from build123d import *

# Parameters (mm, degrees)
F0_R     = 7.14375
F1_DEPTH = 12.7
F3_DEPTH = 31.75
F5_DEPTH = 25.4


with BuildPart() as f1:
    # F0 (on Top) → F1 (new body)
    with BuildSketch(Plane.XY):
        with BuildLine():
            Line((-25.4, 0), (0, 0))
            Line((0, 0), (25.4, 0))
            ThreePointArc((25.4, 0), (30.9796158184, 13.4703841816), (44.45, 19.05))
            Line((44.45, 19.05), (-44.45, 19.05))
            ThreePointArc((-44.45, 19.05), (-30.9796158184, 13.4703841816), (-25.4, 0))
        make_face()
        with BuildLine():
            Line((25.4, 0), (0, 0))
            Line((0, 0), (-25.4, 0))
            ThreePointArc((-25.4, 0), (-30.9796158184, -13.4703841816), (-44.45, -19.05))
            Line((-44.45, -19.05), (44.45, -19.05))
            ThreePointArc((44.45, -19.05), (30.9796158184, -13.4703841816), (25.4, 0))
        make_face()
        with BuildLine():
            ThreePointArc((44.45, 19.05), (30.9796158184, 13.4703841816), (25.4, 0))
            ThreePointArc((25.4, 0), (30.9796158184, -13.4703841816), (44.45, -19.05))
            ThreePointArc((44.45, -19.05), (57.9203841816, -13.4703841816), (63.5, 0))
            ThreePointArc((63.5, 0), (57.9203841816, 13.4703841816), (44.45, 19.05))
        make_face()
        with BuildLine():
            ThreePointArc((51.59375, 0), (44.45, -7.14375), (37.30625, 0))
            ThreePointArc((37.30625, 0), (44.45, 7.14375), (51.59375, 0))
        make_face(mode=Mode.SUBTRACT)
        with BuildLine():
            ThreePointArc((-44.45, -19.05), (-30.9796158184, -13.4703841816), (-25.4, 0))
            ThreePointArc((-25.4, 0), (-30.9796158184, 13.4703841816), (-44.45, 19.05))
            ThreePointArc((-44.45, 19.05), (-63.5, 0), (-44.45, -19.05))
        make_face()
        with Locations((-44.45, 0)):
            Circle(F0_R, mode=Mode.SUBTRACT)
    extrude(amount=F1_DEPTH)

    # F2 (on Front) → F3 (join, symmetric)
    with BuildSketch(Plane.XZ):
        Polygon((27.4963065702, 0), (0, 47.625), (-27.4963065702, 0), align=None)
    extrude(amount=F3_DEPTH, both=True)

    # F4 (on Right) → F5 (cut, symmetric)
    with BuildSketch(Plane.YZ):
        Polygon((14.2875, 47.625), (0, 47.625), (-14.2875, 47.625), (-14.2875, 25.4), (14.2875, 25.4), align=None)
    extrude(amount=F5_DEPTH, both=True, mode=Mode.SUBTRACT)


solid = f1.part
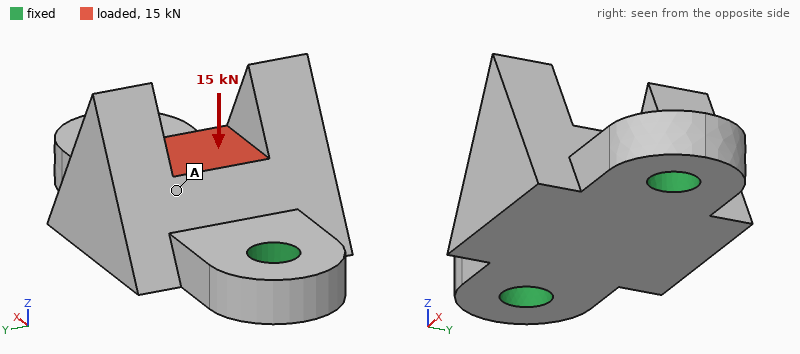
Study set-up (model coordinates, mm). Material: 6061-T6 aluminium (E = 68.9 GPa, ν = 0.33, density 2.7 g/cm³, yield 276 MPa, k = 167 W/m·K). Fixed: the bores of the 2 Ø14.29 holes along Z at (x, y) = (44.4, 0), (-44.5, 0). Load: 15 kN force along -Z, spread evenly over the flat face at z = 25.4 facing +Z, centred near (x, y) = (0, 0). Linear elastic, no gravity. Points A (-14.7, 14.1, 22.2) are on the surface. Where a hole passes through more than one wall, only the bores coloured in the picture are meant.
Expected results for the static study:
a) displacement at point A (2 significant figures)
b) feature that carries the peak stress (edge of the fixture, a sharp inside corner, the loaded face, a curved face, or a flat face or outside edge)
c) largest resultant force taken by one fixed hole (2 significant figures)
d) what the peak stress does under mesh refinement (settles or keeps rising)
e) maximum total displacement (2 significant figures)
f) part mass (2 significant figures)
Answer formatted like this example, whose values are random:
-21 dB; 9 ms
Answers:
45 µm; edge of the fixture; 8.0 kN; keeps rising; 50 µm; 280 g
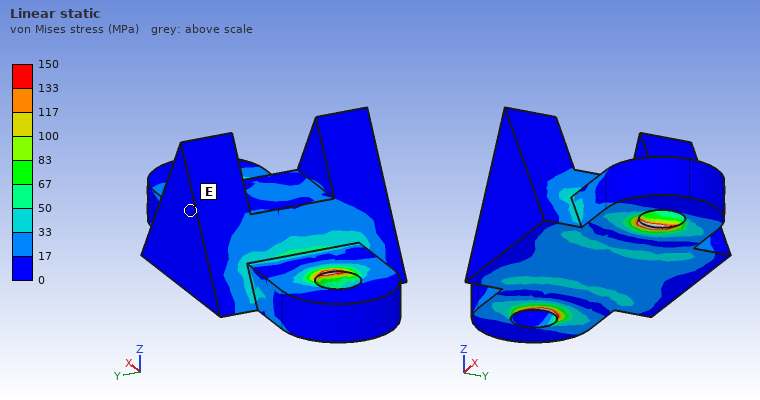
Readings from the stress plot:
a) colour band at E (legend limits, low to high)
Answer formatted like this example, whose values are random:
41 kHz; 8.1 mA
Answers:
0 to 17 MPa
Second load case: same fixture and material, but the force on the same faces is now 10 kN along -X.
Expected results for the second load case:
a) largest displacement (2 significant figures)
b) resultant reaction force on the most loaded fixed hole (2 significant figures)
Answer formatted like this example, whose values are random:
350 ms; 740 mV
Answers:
28 µm; 5.8 kN
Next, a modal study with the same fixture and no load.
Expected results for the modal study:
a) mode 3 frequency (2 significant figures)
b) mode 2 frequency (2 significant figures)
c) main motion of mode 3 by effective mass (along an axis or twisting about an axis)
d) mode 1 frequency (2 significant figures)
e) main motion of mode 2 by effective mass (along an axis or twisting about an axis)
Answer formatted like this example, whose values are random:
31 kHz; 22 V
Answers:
10000 Hz; 6200 Hz; along Y; 3700 Hz; along Z
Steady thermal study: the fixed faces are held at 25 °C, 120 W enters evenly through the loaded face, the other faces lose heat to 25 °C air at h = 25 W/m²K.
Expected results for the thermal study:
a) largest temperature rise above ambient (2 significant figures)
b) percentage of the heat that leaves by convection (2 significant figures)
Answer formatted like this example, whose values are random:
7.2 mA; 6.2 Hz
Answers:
30 K; 5.0 %
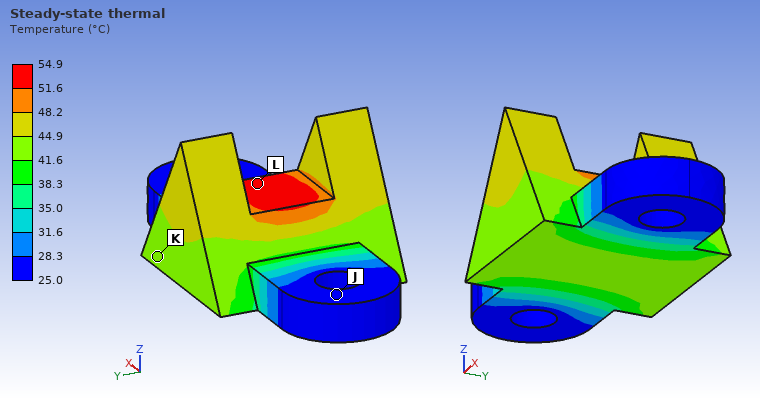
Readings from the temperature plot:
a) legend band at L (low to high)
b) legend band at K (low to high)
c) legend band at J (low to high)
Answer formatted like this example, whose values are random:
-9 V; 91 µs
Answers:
51.6 to 54.9 °C; 41.6 to 44.9 °C; 25.0 to 28.3 °C
